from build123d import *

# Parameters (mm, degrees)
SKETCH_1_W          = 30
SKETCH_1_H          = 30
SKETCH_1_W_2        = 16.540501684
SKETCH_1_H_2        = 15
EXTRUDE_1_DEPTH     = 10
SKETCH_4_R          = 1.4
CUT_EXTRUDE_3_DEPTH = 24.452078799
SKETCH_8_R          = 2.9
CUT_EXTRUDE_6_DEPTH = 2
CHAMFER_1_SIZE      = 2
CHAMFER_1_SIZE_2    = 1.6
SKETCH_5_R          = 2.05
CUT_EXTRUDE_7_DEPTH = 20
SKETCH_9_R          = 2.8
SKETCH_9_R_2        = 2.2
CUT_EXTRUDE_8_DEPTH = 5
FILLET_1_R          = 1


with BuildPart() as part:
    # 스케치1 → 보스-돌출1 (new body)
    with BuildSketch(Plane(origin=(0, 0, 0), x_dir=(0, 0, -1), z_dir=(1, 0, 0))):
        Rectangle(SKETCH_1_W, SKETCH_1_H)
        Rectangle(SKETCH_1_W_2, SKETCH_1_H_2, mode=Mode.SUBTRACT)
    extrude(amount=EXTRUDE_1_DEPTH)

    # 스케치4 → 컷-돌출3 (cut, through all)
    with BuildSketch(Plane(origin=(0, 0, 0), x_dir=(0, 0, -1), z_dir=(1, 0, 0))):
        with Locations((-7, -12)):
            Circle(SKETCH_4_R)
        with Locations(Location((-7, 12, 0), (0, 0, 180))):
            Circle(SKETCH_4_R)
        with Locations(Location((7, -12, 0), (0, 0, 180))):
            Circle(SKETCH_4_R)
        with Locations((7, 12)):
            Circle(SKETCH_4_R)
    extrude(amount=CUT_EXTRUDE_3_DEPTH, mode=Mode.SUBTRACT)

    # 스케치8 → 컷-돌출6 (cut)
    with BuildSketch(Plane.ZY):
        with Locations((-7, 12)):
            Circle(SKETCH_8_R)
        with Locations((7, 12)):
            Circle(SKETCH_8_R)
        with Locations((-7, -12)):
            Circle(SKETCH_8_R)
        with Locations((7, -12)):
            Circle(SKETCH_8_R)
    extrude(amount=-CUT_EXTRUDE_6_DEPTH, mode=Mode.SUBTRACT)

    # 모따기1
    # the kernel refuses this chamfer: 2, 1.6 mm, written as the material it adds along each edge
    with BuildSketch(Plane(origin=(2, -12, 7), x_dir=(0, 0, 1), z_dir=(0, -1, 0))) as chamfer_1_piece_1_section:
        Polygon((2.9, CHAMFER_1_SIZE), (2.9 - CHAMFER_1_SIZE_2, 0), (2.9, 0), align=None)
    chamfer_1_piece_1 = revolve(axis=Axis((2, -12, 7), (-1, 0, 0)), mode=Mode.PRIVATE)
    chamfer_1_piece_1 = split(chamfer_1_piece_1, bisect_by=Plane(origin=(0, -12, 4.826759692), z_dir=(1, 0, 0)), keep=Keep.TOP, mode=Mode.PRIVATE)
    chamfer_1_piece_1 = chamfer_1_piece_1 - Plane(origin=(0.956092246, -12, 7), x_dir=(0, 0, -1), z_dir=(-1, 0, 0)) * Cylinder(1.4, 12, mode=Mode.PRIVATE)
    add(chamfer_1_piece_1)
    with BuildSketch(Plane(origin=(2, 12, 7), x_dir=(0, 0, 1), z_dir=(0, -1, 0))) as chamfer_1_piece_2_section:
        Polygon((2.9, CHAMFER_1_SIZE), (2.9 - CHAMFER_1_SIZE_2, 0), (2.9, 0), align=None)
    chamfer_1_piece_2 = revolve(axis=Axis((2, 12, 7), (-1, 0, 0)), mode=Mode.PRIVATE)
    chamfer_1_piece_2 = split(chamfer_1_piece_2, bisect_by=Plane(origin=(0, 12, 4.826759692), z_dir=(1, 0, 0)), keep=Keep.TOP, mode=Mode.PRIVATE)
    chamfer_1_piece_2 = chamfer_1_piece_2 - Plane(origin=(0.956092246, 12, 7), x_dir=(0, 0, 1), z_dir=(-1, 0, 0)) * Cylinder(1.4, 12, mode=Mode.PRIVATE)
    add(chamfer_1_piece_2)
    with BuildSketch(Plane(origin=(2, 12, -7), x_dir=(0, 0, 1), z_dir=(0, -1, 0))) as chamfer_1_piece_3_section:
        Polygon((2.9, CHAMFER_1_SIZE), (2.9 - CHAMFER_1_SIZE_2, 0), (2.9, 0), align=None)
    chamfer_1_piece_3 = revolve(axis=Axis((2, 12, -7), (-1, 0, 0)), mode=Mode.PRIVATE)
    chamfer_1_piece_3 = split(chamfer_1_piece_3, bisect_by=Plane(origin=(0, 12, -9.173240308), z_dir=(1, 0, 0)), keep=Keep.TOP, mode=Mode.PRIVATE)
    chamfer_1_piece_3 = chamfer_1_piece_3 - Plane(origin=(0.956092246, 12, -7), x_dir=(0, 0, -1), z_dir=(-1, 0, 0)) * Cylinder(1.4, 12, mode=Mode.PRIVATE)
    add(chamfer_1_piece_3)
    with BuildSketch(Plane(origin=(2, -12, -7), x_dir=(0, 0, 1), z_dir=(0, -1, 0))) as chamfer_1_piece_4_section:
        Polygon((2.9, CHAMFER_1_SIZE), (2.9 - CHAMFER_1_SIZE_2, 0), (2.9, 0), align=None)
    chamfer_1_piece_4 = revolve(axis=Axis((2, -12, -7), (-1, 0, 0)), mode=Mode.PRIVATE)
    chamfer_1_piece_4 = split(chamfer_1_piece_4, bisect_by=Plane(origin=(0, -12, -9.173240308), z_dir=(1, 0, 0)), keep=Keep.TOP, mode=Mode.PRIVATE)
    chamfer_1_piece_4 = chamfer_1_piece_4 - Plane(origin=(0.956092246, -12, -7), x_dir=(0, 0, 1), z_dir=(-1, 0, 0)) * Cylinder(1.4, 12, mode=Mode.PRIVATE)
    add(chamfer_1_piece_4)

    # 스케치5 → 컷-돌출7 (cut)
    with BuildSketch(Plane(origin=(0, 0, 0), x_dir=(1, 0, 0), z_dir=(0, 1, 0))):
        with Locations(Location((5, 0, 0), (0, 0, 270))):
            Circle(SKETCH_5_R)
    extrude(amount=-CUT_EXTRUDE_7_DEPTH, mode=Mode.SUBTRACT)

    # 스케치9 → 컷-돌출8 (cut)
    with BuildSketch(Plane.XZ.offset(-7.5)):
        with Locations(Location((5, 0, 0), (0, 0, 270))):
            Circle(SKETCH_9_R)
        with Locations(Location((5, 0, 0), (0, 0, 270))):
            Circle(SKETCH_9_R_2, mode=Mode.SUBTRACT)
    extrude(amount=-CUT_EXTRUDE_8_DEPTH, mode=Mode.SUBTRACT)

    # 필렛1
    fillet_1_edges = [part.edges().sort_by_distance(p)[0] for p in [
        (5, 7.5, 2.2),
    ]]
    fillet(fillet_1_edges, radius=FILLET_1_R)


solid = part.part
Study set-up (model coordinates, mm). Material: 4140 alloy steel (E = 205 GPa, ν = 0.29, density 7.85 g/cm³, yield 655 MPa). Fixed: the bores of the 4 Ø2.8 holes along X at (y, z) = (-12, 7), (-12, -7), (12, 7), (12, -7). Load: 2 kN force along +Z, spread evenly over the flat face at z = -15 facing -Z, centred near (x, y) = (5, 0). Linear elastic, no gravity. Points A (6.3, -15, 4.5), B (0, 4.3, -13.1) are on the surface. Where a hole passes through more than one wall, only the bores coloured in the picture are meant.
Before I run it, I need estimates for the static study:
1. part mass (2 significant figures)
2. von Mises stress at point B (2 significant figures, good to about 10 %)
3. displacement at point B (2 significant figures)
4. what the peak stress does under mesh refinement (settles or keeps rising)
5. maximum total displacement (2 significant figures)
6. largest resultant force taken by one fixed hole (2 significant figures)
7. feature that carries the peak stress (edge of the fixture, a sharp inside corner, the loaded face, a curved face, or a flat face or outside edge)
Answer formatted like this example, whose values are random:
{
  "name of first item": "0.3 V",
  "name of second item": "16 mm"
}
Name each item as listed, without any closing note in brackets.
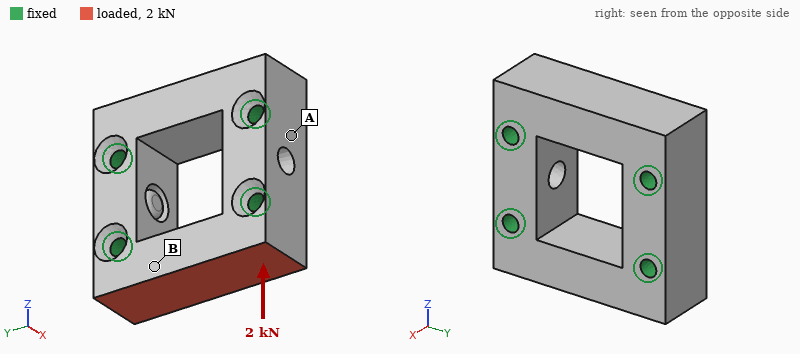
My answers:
{
  "part mass": "48 g",
  "von Mises stress at point B": "14 MPa",
  "displacement at point B": "1.5 µm",
  "what the peak stress does under mesh refinement": "keeps rising",
  "maximum total displacement": "1.9 µm",
  "largest resultant force taken by one fixed hole": "1000 N",
  "feature that carries the peak stress": "edge of the fixture"
}
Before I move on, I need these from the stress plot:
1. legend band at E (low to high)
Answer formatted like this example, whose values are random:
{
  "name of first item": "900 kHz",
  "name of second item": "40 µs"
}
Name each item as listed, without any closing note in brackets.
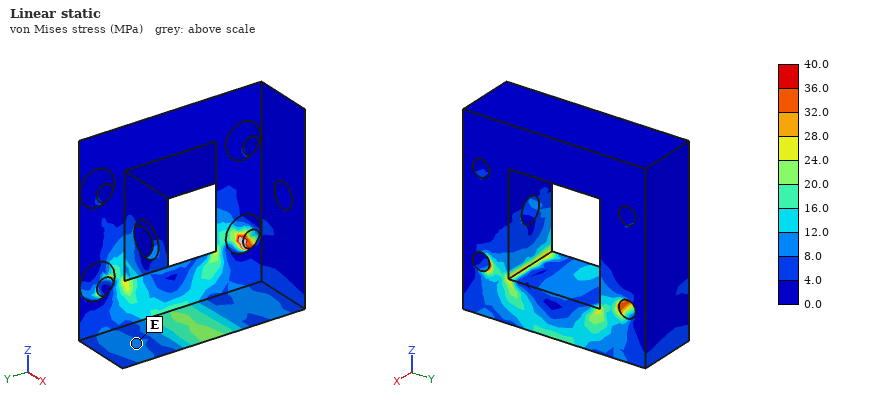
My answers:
{
  "legend band at E": "8.0 to 12.0 MPa"
}
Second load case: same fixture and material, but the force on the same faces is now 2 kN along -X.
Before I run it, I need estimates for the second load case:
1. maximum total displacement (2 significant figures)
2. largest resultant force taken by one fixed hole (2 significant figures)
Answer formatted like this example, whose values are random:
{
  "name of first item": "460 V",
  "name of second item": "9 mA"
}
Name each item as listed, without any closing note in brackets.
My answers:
{
  "maximum total displacement": "5.5 µm",
  "largest resultant force taken by one fixed hole": "1.1 kN"
}
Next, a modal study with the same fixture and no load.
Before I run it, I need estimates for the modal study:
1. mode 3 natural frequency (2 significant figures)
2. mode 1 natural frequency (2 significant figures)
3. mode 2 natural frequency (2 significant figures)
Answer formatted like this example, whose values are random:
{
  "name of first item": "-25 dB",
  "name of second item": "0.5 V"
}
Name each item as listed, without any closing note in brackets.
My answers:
{
  "mode 3 natural frequency": "48 kHz",
  "mode 1 natural frequency": "39 kHz",
  "mode 2 natural frequency": "39 kHz"
}
